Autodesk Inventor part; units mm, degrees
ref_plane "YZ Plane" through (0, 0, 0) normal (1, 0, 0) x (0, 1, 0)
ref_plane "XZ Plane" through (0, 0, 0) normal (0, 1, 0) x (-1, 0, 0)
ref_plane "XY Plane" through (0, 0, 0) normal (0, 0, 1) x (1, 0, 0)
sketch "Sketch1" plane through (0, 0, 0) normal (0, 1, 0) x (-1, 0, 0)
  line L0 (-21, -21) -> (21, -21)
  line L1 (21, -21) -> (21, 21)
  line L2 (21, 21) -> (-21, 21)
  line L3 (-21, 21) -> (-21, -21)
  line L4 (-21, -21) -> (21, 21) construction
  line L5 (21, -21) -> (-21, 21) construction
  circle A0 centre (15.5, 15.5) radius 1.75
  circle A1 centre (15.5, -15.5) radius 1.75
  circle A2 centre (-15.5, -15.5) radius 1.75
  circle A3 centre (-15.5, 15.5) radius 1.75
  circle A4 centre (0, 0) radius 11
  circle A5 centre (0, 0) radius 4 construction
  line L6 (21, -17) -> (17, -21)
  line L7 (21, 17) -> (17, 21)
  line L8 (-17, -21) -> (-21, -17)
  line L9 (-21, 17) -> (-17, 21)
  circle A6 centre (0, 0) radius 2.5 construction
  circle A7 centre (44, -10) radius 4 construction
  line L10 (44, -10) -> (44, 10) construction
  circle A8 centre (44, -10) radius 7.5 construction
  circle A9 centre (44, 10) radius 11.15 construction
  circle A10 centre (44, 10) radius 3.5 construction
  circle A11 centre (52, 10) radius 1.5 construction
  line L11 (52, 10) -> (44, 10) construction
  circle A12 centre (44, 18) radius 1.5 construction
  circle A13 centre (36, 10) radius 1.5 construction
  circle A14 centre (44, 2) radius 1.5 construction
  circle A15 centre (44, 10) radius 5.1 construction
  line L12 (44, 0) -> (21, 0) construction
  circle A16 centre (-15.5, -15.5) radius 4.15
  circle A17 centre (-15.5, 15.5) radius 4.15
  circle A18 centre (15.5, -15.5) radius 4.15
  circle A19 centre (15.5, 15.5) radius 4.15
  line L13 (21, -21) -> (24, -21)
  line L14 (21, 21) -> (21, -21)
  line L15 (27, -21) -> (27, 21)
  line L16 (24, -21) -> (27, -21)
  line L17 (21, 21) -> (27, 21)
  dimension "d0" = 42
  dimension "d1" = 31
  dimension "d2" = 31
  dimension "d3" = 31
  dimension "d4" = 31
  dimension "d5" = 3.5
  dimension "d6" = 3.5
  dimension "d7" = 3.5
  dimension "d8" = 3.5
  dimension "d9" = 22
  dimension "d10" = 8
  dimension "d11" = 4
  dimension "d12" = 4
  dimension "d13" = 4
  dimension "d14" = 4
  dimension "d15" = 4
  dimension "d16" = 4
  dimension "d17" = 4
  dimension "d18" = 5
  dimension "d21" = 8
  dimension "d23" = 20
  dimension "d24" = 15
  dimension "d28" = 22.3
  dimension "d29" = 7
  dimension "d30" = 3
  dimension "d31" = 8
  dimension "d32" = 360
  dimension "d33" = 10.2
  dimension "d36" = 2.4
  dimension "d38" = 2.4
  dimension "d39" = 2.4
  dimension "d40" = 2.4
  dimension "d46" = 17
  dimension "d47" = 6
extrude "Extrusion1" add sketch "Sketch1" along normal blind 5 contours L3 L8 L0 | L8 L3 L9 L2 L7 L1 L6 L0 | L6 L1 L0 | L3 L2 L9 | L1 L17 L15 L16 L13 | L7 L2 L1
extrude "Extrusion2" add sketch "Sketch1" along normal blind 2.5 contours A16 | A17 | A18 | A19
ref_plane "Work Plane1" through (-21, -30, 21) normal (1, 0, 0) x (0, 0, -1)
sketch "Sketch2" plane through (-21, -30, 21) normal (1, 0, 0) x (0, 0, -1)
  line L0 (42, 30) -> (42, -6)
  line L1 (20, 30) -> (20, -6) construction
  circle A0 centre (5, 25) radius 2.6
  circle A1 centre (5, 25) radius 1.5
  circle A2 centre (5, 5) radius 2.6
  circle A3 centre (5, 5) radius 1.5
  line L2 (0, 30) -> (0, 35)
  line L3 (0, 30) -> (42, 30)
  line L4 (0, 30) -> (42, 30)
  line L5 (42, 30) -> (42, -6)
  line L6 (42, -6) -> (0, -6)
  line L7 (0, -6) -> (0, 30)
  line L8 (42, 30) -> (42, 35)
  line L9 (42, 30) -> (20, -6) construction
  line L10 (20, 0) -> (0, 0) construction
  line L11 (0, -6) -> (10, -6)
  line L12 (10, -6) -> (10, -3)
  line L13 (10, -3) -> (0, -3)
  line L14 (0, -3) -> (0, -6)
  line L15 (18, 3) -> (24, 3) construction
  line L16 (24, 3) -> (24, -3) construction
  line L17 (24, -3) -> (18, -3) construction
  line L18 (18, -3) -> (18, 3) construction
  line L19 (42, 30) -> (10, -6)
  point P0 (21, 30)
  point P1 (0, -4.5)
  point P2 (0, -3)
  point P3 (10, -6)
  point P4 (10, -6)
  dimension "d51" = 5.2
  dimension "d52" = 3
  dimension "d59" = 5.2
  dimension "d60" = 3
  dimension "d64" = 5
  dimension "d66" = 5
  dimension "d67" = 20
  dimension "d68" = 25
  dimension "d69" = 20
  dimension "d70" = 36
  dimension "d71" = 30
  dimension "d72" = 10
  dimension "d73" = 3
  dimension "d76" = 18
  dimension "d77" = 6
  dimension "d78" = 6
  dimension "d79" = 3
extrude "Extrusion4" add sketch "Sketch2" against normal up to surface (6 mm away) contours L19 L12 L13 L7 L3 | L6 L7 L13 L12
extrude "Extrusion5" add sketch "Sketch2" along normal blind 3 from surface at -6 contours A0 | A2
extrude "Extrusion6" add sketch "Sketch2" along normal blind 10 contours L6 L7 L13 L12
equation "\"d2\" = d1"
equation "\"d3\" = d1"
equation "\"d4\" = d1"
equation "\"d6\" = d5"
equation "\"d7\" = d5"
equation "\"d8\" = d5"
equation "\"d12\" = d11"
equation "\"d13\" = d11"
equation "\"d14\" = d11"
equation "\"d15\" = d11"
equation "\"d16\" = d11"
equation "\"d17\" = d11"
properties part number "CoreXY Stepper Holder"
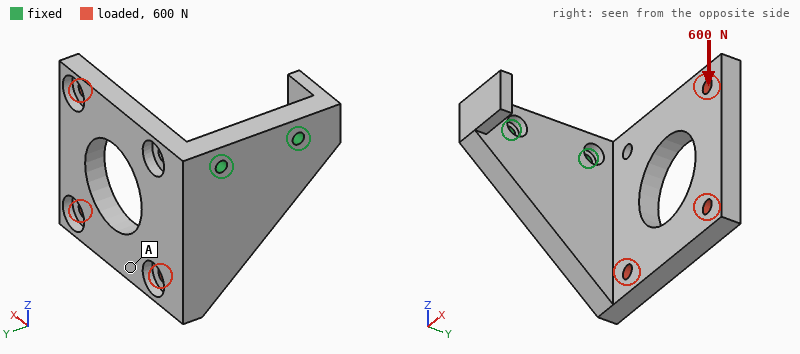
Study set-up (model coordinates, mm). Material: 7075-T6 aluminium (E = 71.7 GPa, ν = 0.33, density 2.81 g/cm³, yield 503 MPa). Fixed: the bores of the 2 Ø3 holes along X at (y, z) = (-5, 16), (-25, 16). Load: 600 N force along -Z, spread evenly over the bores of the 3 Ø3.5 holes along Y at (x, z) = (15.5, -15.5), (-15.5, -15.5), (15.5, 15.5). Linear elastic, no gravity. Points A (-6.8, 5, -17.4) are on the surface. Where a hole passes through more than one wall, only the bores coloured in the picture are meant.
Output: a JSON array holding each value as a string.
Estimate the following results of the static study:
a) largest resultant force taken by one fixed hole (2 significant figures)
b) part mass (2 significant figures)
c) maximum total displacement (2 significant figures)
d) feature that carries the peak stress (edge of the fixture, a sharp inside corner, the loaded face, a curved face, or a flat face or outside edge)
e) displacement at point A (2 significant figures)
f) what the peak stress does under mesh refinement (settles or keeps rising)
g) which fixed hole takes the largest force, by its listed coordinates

["740 N", "37 g", "0.60 mm", "edge of the fixture", "0.38 mm", "keeps rising", "(-5, 16)"]
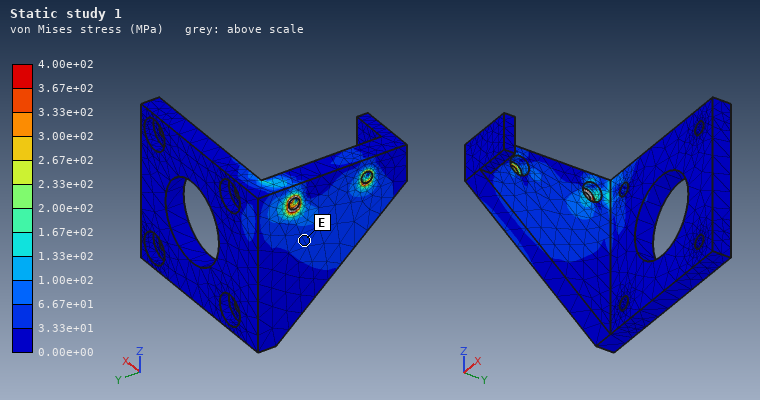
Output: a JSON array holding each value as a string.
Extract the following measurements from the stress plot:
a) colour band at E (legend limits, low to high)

["3.33e+01 to 6.67e+01 MPa"]
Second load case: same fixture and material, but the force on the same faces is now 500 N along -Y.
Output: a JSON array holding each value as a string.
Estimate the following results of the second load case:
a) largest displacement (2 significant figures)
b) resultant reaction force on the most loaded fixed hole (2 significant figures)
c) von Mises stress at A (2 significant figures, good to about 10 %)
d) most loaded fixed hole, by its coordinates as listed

["0.71 mm", "1.1 kN", "58 MPa", "(-25, 16)"]
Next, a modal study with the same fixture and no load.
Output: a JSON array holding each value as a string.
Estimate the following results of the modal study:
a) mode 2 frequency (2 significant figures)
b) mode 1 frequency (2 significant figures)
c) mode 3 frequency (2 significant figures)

["1500 Hz", "1300 Hz", "3800 Hz"]
